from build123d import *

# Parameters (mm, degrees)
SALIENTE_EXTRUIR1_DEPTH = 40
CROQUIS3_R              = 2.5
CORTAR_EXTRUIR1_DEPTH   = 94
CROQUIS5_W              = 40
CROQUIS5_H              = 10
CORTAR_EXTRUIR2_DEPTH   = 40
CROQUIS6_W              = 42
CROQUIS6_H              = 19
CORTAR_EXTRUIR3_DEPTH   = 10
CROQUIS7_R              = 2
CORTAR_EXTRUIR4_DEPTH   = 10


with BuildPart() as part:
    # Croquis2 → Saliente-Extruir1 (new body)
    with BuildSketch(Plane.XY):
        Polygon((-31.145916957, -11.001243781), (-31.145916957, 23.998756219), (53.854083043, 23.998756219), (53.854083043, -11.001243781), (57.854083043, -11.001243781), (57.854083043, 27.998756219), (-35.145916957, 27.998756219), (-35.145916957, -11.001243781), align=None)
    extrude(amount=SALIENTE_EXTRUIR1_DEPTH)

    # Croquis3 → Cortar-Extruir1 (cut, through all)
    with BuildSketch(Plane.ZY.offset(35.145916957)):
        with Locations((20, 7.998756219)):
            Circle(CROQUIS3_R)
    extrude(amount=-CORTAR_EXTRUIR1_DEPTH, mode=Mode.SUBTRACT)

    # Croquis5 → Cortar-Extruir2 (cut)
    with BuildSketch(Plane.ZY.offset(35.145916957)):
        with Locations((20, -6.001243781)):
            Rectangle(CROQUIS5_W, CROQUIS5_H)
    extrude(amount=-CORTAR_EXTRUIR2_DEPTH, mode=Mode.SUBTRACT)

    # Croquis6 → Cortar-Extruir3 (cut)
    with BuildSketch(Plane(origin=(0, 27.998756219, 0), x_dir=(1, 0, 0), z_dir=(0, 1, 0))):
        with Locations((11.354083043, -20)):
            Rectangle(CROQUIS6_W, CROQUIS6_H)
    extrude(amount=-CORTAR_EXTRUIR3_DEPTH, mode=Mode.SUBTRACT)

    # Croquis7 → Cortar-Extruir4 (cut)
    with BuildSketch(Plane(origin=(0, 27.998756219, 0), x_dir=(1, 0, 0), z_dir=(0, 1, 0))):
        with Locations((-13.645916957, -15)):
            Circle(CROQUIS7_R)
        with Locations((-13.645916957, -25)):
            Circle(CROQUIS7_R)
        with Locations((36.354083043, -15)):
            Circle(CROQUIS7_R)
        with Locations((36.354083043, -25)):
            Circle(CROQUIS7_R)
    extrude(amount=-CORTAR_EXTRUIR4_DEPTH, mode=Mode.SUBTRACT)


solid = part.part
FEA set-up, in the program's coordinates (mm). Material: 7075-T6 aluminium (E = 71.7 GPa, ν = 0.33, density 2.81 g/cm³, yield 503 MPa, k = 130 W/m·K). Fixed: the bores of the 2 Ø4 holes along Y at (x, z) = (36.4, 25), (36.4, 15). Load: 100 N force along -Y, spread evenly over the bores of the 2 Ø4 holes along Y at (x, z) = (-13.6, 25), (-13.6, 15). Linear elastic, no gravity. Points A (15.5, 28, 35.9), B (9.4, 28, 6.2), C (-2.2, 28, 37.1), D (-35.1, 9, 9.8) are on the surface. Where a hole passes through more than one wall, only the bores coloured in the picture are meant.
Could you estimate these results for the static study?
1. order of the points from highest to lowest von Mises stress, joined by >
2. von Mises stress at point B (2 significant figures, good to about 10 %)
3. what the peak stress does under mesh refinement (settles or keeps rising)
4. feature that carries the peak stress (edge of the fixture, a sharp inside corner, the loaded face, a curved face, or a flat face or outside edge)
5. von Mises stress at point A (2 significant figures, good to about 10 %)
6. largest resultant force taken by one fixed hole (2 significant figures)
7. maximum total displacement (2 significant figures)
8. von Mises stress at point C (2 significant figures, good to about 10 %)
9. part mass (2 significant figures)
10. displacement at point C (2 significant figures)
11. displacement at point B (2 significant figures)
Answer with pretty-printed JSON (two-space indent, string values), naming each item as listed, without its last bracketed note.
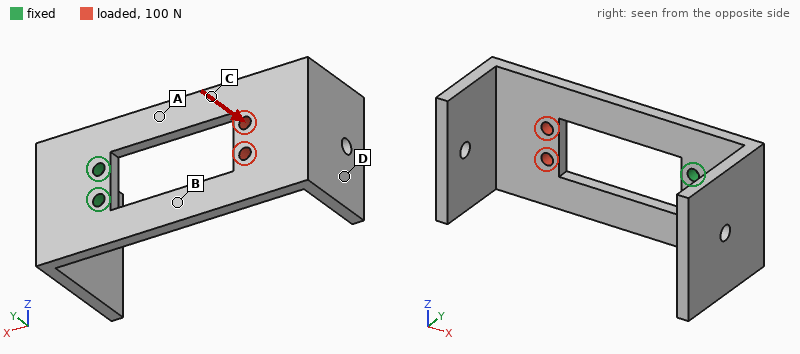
{
  "order of the points from highest to lowest von Mises stress, joined by >": "A > B > C > D",
  "von Mises stress at point B": "42 MPa",
  "what the peak stress does under mesh refinement": "keeps rising",
  "feature that carries the peak stress": "edge of the fixture",
  "von Mises stress at point A": "52 MPa",
  "largest resultant force taken by one fixed hole": "50 N",
  "maximum total displacement": "1.1 mm",
  "von Mises stress at point C": "21 MPa",
  "part mass": "59 g",
  "displacement at point C": "0.42 mm",
  "displacement at point B": "0.24 mm"
}
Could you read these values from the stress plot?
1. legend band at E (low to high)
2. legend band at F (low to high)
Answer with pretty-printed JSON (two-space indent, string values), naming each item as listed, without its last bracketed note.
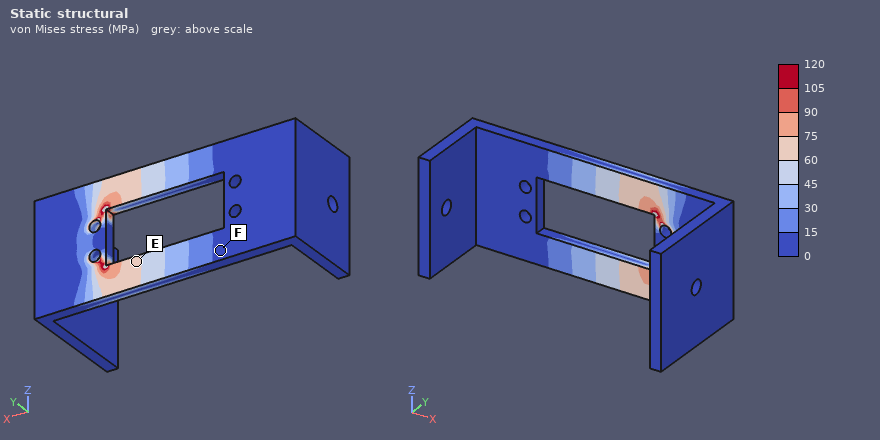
{
  "legend band at E": "60 to 75 MPa",
  "legend band at F": "0 to 15 MPa"
}
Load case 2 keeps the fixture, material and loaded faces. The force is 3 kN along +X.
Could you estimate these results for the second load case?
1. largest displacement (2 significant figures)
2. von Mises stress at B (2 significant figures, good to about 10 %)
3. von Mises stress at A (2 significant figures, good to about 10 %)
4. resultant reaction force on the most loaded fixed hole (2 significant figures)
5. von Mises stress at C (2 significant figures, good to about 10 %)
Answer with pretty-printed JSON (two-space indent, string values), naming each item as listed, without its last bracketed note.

{
  "largest displacement": "48 µm",
  "von Mises stress at B": "38 MPa",
  "von Mises stress at A": "33 MPa",
  "resultant reaction force on the most loaded fixed hole": "1.6 kN",
  "von Mises stress at C": "29 MPa"
}
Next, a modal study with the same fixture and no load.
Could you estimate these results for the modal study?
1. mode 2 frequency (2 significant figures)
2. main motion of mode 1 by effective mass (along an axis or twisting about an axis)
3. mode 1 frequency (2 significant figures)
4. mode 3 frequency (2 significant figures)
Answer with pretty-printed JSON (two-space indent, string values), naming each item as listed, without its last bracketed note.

{
  "mode 2 frequency": "860 Hz",
  "main motion of mode 1 by effective mass": "along Y",
  "mode 1 frequency": "280 Hz",
  "mode 3 frequency": "1300 Hz"
}
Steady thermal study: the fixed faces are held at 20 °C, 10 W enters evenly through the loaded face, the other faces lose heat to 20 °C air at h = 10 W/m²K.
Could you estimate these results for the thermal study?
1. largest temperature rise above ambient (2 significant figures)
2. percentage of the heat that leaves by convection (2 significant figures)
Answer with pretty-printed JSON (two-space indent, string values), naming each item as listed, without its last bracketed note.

{
  "largest temperature rise above ambient": "46 K",
  "percentage of the heat that leaves by convection": "25 %"
}
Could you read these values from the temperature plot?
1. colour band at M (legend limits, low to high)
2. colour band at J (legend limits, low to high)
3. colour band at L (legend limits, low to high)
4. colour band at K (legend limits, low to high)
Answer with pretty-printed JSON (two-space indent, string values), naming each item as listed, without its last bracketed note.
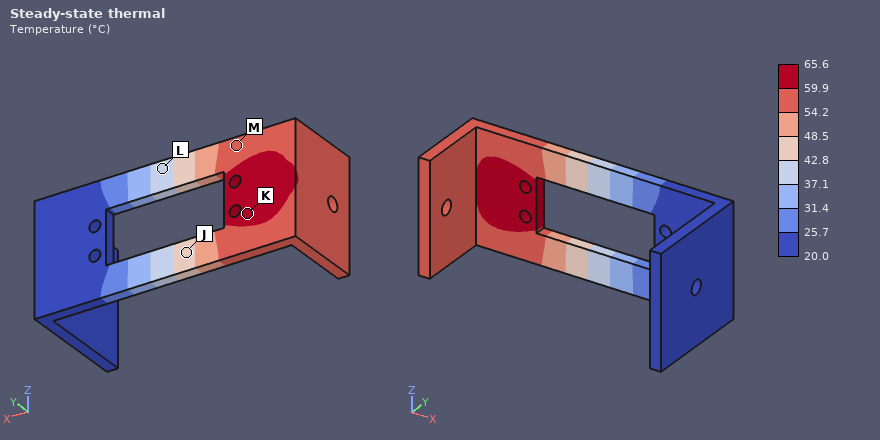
{
  "colour band at M": "54.2 to 59.9 °C",
  "colour band at J": "42.8 to 48.5 °C",
  "colour band at L": "37.1 to 42.8 °C",
  "colour band at K": "59.9 to 65.6 °C"
}
